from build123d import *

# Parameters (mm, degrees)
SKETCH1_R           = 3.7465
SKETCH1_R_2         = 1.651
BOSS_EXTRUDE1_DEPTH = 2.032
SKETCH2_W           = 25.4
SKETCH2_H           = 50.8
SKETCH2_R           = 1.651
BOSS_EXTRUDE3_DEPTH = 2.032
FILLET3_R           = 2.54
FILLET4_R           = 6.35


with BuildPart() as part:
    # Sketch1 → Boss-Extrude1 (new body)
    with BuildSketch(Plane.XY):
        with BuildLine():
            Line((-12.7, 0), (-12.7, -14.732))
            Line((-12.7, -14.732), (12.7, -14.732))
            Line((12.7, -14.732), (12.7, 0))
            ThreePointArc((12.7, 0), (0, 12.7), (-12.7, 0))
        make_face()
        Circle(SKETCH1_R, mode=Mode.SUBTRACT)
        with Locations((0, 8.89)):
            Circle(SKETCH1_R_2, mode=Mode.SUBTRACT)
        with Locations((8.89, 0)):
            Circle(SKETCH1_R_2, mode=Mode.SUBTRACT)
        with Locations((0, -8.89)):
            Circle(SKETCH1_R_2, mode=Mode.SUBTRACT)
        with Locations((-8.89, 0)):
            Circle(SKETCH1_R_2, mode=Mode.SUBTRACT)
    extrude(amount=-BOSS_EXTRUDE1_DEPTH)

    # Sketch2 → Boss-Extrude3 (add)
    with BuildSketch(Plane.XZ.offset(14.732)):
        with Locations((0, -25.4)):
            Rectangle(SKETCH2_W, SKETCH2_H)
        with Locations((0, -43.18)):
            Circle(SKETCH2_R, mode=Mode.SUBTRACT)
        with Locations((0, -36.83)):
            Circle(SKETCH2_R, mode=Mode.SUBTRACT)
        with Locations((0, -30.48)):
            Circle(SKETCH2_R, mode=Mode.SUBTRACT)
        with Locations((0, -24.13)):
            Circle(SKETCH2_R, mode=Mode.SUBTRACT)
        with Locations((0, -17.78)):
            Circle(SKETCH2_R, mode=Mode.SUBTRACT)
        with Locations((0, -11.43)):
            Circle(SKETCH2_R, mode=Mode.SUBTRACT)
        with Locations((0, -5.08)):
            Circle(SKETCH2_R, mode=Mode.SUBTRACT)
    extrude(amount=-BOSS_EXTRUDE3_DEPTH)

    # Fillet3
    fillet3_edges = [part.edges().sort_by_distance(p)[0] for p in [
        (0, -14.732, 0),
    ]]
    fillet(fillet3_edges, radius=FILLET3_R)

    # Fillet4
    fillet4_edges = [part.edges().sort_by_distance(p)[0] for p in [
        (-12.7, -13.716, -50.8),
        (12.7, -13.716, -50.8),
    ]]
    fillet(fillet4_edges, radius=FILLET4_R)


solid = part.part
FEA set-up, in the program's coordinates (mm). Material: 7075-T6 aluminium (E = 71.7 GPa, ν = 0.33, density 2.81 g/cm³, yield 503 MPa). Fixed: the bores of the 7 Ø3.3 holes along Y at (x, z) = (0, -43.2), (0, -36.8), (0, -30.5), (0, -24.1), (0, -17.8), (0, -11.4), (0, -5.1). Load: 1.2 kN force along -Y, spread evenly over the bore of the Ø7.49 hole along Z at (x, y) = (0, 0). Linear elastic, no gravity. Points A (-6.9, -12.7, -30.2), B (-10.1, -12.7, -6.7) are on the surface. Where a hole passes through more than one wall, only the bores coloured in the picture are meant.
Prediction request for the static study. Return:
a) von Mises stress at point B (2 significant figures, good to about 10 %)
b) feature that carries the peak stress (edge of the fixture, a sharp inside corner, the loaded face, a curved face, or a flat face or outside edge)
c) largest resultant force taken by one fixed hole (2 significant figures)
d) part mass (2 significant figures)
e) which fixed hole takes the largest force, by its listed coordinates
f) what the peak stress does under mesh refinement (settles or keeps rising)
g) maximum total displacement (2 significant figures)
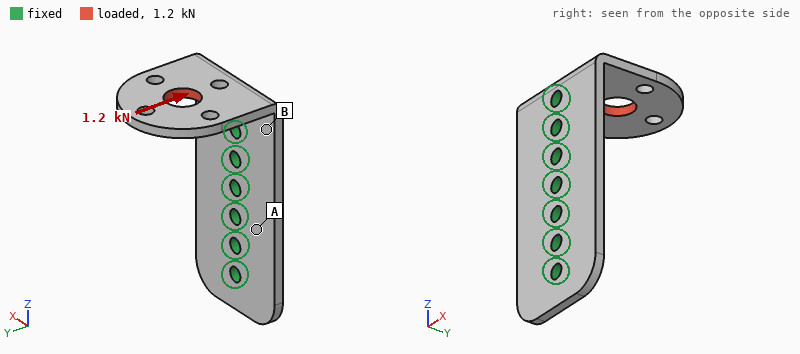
50 MPa
edge of the fixture
1.3 kN
9.7 g
(0, -5.1)
keeps rising
0.23 mm
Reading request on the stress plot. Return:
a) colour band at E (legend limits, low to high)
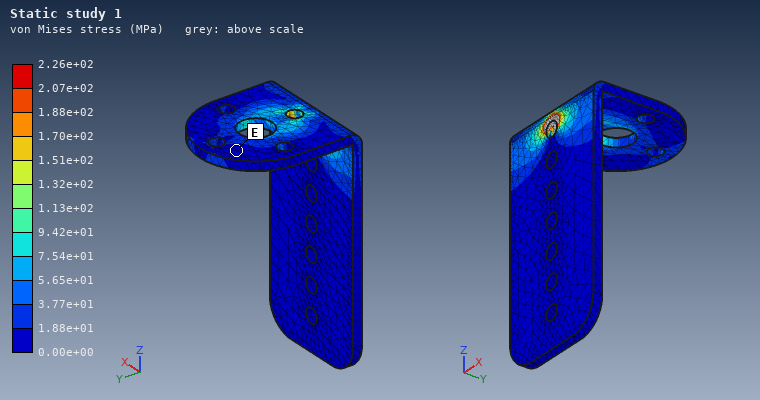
0.00e+00 to 1.88e+01 MPa
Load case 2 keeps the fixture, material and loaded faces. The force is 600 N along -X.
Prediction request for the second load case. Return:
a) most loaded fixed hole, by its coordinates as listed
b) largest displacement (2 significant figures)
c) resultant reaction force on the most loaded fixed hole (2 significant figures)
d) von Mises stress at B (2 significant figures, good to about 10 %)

(0, -5.1)
0.44 mm
600 N
110 MPa
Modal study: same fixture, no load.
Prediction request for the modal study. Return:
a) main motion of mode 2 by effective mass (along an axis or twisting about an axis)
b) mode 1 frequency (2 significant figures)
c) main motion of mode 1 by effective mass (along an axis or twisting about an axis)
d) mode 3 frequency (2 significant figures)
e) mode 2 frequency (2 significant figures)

along X
2300 Hz
along Z
6700 Hz
4000 Hz
